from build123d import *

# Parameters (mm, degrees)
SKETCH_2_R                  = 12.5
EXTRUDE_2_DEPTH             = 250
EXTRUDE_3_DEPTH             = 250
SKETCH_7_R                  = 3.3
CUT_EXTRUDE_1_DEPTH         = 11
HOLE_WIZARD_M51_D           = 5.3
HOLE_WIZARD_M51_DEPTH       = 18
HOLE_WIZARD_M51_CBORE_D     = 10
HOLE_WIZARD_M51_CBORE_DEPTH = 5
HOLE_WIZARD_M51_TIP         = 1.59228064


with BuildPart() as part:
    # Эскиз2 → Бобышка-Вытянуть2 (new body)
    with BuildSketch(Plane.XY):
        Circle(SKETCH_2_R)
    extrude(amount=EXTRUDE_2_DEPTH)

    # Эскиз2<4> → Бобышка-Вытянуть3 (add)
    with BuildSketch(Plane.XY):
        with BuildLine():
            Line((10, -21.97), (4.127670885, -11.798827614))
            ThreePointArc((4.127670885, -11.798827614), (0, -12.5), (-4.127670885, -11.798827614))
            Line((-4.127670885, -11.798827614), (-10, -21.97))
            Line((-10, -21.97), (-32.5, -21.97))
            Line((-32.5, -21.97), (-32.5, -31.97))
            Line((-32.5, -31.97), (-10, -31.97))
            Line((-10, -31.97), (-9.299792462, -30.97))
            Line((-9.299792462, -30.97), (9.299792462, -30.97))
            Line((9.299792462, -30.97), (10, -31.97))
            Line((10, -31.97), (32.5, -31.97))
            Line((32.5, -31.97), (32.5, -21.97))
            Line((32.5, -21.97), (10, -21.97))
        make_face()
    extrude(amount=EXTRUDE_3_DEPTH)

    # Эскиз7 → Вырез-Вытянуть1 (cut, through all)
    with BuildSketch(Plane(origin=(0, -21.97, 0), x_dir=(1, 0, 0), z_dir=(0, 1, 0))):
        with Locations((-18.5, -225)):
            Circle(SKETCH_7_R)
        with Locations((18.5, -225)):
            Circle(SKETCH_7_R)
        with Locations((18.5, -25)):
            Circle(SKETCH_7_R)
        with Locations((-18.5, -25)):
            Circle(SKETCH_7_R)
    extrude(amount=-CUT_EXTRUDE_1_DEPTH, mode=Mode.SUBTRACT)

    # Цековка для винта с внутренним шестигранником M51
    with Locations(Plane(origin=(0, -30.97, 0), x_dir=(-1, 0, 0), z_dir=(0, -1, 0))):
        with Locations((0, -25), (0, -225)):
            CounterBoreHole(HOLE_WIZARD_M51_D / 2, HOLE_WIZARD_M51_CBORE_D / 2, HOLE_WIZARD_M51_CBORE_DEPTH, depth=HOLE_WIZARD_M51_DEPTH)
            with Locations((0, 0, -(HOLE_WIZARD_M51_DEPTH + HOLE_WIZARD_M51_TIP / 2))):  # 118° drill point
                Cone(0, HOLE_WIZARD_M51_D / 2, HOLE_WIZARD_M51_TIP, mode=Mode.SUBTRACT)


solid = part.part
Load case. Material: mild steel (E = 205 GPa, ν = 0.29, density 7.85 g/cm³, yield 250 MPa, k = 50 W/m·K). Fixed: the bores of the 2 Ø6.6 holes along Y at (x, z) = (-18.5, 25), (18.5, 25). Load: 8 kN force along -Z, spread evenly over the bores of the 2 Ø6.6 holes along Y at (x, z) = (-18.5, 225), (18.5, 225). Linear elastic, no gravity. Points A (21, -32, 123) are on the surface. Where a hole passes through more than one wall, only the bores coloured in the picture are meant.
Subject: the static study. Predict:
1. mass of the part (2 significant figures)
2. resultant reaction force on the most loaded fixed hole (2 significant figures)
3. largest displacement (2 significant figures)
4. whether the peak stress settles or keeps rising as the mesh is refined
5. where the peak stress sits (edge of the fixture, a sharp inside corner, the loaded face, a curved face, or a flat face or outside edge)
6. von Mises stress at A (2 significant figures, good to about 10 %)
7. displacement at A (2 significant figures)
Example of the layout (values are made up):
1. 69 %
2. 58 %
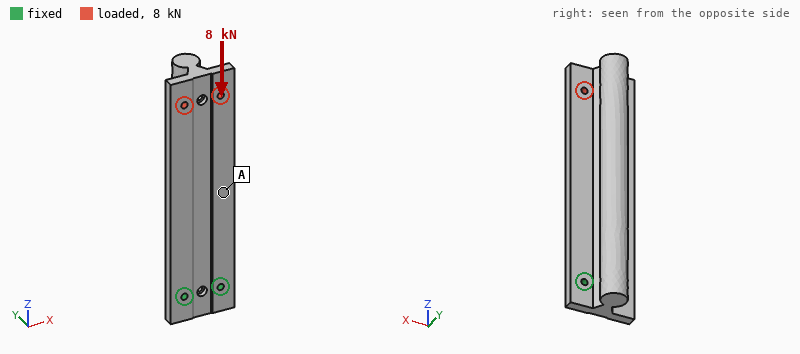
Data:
1. 2.5 kg
2. 4.0 kN
3. 48 µm
4. keeps rising
5. edge of the fixture
6. 13 MPa
7. 10 µm
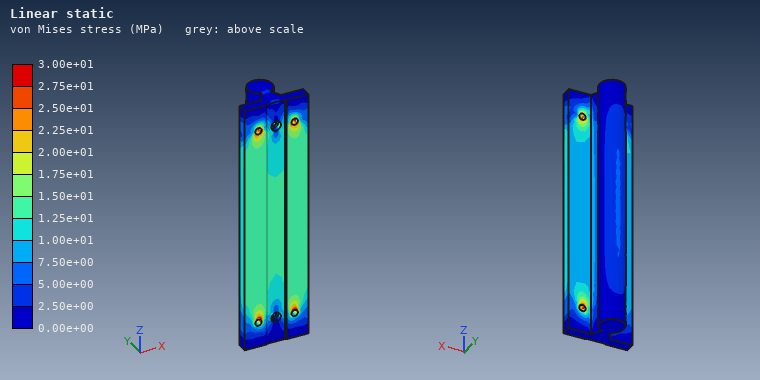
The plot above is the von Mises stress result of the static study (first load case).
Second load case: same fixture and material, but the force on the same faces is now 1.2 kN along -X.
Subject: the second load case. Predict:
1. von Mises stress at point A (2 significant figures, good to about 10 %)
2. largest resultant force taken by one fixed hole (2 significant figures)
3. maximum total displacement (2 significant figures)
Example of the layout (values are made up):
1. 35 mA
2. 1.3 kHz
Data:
1. 11 MPa
2. 6.0 kN
3. 90 µm
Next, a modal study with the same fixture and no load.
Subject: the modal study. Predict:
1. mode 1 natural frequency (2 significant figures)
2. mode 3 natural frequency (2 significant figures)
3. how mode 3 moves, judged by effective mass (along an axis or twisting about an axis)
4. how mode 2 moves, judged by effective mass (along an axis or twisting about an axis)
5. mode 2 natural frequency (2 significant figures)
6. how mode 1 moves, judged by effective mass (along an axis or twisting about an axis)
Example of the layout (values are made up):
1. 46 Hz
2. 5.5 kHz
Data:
1. 290 Hz
2. 1400 Hz
3. twisting about Z
4. along X
5. 690 Hz
6. along Y
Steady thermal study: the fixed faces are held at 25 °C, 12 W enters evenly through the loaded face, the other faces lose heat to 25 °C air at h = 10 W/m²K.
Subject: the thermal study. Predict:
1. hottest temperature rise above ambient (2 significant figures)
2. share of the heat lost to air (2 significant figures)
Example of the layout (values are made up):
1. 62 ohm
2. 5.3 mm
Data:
1. 28 K
2. 57 %
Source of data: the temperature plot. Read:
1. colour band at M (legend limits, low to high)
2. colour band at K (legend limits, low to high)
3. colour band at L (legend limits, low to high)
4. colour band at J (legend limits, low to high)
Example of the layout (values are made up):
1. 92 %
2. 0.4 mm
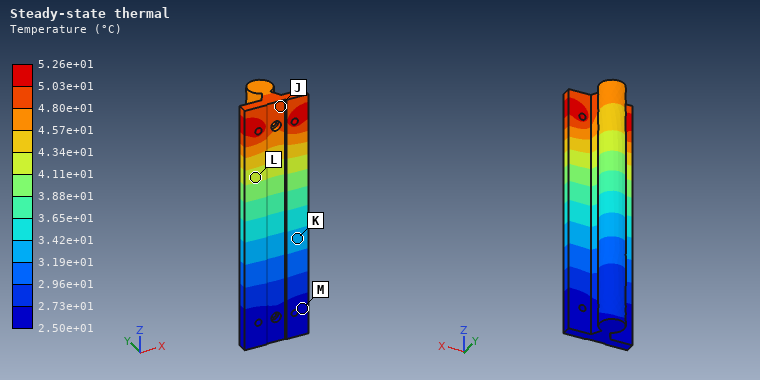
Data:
1. 2.50e+01 to 2.73e+01 °C
2. 3.19e+01 to 3.42e+01 °C
3. 4.11e+01 to 4.34e+01 °C
4. 4.80e+01 to 5.03e+01 °C
